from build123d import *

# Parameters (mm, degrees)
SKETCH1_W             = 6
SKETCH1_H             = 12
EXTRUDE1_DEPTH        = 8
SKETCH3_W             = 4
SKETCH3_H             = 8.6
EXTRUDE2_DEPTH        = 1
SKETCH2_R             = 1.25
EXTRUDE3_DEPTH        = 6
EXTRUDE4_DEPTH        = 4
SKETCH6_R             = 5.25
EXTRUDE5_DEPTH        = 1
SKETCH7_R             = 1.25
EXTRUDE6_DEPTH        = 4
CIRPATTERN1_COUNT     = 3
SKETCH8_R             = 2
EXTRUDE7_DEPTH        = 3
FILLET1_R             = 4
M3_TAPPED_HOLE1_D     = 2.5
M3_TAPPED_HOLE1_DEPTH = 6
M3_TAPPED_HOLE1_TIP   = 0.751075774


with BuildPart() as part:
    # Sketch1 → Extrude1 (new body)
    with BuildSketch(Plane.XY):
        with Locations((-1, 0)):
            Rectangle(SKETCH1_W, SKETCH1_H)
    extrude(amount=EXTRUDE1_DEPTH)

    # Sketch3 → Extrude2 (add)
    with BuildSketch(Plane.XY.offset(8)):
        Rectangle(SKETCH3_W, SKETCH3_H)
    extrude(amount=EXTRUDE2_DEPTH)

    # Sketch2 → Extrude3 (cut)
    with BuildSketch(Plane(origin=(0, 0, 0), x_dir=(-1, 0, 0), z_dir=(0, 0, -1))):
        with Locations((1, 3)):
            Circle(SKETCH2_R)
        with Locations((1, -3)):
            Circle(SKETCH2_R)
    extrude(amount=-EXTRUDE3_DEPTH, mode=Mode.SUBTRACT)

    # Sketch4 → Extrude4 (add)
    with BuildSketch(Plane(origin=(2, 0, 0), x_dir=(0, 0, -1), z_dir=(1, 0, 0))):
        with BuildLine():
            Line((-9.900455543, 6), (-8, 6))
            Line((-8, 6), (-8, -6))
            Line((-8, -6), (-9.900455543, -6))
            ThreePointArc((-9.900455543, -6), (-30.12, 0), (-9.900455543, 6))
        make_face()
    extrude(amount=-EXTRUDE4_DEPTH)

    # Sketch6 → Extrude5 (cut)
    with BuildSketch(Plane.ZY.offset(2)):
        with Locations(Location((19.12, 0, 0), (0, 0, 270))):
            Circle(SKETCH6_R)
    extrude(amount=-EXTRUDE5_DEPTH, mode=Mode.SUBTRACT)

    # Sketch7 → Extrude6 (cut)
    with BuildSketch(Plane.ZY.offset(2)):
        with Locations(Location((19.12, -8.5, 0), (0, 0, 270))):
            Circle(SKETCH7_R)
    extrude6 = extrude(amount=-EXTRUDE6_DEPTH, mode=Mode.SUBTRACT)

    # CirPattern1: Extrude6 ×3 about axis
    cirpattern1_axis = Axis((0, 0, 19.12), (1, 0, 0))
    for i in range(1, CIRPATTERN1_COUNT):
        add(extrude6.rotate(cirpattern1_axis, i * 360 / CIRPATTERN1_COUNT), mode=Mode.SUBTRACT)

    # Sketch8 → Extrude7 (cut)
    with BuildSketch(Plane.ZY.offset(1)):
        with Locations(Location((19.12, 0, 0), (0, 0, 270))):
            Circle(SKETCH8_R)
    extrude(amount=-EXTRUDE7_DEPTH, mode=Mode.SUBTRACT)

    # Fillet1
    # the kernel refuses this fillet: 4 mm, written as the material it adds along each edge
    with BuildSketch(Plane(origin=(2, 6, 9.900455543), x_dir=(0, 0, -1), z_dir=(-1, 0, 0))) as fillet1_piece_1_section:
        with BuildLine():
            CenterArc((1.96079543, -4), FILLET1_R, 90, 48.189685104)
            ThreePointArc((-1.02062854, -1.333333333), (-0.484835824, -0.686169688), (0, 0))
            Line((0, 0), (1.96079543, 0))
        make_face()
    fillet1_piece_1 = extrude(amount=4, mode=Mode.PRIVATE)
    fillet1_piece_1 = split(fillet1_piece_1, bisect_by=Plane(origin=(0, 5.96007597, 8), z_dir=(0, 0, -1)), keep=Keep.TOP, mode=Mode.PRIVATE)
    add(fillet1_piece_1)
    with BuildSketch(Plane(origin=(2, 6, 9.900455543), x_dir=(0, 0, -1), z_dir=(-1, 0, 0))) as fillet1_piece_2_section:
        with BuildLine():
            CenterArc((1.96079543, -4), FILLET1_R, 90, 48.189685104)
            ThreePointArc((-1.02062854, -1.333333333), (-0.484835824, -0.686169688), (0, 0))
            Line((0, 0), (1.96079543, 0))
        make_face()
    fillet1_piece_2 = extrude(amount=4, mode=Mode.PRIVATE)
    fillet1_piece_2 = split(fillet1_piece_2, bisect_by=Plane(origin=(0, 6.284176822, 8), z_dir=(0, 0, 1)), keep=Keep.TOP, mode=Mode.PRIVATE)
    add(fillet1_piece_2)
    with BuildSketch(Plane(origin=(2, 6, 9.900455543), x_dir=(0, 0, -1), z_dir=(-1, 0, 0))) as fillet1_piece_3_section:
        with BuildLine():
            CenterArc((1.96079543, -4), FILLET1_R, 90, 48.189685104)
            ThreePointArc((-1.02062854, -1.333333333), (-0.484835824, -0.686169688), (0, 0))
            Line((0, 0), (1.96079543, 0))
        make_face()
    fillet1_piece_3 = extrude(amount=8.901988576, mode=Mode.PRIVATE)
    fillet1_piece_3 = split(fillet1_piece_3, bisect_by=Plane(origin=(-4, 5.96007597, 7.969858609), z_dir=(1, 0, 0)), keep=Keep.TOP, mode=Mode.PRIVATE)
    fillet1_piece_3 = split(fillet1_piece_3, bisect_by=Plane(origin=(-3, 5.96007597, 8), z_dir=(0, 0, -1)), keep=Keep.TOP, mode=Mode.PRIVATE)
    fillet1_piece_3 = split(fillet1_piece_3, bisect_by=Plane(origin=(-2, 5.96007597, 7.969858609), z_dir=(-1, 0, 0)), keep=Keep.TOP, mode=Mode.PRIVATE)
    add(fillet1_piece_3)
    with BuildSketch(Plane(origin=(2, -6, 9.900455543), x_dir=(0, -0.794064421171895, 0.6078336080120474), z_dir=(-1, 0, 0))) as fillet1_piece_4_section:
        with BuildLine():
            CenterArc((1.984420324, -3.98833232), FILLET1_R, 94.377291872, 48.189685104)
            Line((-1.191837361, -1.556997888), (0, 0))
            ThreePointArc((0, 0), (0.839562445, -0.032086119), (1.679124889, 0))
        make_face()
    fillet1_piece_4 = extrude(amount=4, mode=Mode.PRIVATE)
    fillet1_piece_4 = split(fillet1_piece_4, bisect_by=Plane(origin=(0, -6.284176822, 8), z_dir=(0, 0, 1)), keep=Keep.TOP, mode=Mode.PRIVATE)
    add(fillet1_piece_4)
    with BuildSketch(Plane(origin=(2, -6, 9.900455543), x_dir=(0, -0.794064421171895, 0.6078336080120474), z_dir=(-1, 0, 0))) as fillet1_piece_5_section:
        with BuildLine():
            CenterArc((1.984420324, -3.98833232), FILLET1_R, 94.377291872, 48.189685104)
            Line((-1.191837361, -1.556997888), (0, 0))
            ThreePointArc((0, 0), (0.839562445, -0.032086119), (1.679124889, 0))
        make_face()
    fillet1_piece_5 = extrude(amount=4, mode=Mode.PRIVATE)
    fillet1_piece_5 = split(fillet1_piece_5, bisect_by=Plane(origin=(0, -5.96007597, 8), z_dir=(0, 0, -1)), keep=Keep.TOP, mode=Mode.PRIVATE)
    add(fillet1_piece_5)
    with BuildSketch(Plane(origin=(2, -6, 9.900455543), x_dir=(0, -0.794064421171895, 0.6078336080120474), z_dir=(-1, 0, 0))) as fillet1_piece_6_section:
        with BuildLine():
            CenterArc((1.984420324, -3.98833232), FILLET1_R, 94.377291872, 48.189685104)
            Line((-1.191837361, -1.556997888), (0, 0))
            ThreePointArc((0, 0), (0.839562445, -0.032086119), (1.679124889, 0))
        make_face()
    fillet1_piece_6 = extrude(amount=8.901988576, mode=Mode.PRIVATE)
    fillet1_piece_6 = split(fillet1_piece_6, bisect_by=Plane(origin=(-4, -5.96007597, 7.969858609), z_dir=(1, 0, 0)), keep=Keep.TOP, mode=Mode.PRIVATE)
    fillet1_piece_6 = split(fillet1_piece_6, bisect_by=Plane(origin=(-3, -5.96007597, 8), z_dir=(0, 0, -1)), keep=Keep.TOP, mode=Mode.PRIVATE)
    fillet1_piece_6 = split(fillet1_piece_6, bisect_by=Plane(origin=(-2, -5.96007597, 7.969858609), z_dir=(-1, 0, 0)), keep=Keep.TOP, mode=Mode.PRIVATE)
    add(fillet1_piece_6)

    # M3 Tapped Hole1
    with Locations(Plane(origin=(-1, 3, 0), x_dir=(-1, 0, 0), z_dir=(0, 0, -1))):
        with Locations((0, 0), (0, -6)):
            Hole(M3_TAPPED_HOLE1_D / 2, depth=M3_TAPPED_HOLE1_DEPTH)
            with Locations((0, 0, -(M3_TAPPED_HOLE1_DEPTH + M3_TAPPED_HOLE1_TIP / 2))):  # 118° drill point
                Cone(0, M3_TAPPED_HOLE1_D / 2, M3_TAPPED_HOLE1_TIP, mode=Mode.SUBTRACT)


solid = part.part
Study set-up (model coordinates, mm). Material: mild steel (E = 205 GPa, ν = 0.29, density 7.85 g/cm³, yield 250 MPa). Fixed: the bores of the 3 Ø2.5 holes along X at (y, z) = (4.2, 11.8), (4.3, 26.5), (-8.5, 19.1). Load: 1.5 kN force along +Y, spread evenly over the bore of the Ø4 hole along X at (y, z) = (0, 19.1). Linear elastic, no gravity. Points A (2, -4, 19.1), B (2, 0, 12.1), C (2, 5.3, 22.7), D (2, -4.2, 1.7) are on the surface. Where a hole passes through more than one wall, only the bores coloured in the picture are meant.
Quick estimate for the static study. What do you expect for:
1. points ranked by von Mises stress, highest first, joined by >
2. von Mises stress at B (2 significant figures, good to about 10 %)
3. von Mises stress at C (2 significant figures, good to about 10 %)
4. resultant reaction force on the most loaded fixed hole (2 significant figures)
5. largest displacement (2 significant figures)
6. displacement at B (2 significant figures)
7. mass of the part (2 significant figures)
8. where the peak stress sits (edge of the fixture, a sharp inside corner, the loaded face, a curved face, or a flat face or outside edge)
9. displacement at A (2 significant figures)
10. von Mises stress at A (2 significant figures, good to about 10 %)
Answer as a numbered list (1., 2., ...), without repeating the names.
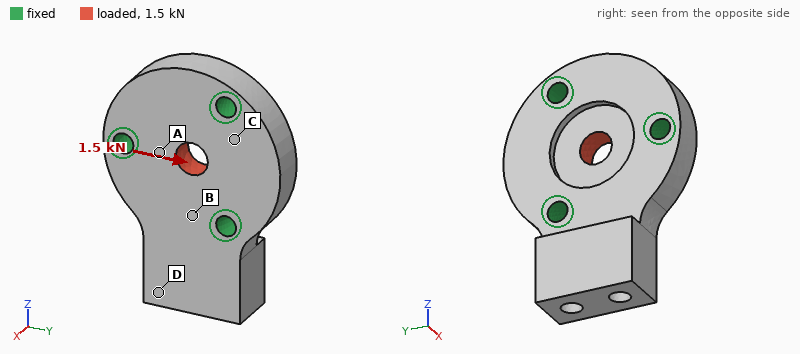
1. A > C > B > D
2. 9.4 MPa
3. 20 MPa
4. 530 N
5. 1.5 µm
6. 0.25 µm
7. 15 g
8. the loaded face
9. 0.63 µm
10. 41 MPa
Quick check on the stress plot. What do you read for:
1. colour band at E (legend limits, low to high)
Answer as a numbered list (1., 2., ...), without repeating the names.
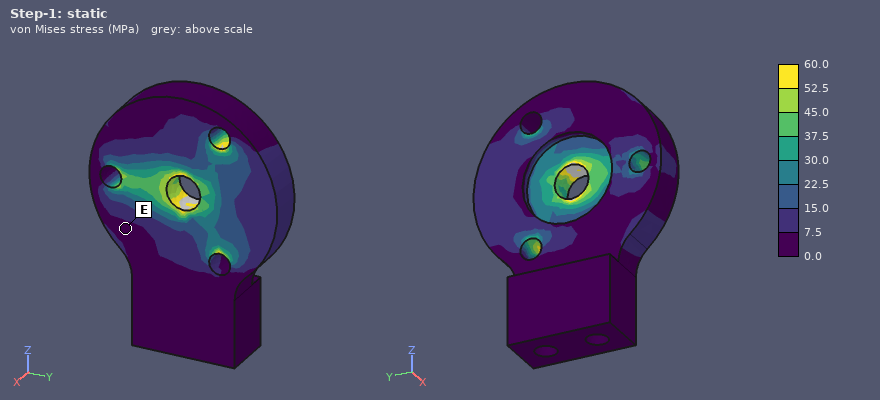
1. 0.0 to 7.5 MPa
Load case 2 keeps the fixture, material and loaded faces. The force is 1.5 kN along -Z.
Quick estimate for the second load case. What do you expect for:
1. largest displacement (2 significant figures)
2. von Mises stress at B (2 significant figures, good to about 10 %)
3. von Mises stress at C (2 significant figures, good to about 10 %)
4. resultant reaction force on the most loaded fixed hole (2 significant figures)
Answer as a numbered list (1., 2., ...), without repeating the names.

1. 1.4 µm
2. 18 MPa
3. 11 MPa
4. 520 N
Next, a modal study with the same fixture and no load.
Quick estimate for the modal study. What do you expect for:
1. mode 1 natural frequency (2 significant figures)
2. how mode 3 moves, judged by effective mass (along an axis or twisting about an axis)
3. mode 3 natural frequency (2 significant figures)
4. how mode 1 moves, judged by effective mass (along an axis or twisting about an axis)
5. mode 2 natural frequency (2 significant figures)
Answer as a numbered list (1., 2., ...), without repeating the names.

1. 16 kHz
2. along Y
3. 39 kHz
4. along X
5. 35 kHz
